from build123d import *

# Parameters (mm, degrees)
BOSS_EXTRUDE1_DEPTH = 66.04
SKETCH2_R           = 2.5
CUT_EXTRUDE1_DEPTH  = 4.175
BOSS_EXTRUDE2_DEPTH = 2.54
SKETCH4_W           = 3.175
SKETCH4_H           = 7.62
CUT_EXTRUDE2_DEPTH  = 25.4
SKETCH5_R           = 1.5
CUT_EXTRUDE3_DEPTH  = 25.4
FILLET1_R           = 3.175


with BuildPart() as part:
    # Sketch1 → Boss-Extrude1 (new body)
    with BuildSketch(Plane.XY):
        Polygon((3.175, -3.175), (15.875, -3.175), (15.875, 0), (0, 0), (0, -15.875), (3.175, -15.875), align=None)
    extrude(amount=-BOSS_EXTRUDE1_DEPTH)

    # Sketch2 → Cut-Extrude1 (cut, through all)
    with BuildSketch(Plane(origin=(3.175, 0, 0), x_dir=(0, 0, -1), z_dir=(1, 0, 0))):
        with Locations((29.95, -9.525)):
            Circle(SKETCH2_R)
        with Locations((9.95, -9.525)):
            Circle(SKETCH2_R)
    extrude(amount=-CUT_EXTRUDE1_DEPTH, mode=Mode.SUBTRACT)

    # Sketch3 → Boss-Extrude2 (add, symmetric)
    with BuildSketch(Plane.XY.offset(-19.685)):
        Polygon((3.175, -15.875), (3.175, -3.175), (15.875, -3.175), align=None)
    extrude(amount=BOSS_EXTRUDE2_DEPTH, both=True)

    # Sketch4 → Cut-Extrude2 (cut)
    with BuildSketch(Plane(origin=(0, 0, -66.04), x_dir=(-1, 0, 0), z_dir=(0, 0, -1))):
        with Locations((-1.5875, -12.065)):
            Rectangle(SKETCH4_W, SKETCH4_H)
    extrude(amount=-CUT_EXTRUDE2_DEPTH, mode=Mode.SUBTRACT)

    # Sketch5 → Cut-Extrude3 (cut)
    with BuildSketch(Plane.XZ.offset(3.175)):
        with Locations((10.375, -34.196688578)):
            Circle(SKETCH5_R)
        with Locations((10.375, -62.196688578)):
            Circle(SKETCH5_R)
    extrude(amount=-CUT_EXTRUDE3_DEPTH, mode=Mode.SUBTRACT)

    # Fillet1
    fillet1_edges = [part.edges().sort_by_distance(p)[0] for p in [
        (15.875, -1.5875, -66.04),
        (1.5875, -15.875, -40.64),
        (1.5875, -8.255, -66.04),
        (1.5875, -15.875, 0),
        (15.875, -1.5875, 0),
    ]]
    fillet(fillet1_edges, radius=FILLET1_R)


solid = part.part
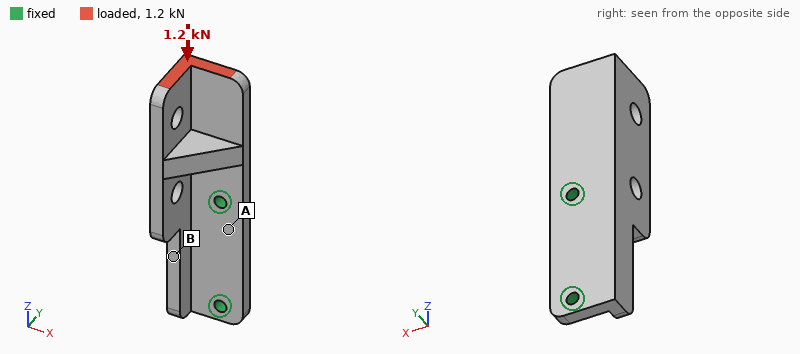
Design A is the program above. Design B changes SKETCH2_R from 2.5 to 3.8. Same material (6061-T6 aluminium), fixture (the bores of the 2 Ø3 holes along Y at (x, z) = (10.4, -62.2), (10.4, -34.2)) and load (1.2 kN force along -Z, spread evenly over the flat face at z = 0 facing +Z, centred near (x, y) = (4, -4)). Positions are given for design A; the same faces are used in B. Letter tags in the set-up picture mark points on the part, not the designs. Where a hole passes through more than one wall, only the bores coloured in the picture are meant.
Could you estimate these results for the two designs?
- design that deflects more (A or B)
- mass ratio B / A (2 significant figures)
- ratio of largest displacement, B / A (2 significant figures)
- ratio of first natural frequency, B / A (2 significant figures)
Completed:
B
0.97
1.2
1.0
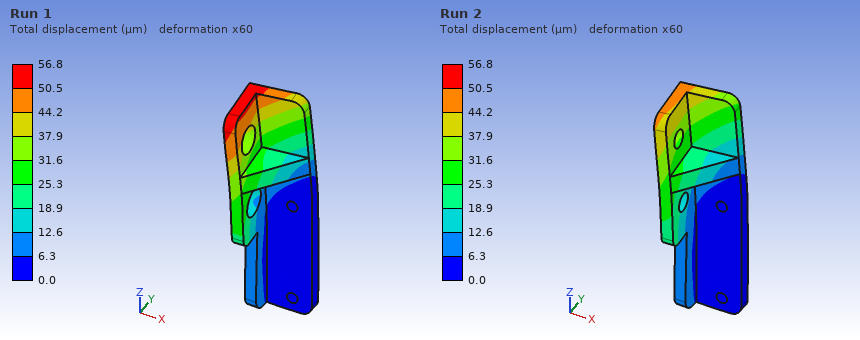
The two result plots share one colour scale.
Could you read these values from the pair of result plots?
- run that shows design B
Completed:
Run 1
